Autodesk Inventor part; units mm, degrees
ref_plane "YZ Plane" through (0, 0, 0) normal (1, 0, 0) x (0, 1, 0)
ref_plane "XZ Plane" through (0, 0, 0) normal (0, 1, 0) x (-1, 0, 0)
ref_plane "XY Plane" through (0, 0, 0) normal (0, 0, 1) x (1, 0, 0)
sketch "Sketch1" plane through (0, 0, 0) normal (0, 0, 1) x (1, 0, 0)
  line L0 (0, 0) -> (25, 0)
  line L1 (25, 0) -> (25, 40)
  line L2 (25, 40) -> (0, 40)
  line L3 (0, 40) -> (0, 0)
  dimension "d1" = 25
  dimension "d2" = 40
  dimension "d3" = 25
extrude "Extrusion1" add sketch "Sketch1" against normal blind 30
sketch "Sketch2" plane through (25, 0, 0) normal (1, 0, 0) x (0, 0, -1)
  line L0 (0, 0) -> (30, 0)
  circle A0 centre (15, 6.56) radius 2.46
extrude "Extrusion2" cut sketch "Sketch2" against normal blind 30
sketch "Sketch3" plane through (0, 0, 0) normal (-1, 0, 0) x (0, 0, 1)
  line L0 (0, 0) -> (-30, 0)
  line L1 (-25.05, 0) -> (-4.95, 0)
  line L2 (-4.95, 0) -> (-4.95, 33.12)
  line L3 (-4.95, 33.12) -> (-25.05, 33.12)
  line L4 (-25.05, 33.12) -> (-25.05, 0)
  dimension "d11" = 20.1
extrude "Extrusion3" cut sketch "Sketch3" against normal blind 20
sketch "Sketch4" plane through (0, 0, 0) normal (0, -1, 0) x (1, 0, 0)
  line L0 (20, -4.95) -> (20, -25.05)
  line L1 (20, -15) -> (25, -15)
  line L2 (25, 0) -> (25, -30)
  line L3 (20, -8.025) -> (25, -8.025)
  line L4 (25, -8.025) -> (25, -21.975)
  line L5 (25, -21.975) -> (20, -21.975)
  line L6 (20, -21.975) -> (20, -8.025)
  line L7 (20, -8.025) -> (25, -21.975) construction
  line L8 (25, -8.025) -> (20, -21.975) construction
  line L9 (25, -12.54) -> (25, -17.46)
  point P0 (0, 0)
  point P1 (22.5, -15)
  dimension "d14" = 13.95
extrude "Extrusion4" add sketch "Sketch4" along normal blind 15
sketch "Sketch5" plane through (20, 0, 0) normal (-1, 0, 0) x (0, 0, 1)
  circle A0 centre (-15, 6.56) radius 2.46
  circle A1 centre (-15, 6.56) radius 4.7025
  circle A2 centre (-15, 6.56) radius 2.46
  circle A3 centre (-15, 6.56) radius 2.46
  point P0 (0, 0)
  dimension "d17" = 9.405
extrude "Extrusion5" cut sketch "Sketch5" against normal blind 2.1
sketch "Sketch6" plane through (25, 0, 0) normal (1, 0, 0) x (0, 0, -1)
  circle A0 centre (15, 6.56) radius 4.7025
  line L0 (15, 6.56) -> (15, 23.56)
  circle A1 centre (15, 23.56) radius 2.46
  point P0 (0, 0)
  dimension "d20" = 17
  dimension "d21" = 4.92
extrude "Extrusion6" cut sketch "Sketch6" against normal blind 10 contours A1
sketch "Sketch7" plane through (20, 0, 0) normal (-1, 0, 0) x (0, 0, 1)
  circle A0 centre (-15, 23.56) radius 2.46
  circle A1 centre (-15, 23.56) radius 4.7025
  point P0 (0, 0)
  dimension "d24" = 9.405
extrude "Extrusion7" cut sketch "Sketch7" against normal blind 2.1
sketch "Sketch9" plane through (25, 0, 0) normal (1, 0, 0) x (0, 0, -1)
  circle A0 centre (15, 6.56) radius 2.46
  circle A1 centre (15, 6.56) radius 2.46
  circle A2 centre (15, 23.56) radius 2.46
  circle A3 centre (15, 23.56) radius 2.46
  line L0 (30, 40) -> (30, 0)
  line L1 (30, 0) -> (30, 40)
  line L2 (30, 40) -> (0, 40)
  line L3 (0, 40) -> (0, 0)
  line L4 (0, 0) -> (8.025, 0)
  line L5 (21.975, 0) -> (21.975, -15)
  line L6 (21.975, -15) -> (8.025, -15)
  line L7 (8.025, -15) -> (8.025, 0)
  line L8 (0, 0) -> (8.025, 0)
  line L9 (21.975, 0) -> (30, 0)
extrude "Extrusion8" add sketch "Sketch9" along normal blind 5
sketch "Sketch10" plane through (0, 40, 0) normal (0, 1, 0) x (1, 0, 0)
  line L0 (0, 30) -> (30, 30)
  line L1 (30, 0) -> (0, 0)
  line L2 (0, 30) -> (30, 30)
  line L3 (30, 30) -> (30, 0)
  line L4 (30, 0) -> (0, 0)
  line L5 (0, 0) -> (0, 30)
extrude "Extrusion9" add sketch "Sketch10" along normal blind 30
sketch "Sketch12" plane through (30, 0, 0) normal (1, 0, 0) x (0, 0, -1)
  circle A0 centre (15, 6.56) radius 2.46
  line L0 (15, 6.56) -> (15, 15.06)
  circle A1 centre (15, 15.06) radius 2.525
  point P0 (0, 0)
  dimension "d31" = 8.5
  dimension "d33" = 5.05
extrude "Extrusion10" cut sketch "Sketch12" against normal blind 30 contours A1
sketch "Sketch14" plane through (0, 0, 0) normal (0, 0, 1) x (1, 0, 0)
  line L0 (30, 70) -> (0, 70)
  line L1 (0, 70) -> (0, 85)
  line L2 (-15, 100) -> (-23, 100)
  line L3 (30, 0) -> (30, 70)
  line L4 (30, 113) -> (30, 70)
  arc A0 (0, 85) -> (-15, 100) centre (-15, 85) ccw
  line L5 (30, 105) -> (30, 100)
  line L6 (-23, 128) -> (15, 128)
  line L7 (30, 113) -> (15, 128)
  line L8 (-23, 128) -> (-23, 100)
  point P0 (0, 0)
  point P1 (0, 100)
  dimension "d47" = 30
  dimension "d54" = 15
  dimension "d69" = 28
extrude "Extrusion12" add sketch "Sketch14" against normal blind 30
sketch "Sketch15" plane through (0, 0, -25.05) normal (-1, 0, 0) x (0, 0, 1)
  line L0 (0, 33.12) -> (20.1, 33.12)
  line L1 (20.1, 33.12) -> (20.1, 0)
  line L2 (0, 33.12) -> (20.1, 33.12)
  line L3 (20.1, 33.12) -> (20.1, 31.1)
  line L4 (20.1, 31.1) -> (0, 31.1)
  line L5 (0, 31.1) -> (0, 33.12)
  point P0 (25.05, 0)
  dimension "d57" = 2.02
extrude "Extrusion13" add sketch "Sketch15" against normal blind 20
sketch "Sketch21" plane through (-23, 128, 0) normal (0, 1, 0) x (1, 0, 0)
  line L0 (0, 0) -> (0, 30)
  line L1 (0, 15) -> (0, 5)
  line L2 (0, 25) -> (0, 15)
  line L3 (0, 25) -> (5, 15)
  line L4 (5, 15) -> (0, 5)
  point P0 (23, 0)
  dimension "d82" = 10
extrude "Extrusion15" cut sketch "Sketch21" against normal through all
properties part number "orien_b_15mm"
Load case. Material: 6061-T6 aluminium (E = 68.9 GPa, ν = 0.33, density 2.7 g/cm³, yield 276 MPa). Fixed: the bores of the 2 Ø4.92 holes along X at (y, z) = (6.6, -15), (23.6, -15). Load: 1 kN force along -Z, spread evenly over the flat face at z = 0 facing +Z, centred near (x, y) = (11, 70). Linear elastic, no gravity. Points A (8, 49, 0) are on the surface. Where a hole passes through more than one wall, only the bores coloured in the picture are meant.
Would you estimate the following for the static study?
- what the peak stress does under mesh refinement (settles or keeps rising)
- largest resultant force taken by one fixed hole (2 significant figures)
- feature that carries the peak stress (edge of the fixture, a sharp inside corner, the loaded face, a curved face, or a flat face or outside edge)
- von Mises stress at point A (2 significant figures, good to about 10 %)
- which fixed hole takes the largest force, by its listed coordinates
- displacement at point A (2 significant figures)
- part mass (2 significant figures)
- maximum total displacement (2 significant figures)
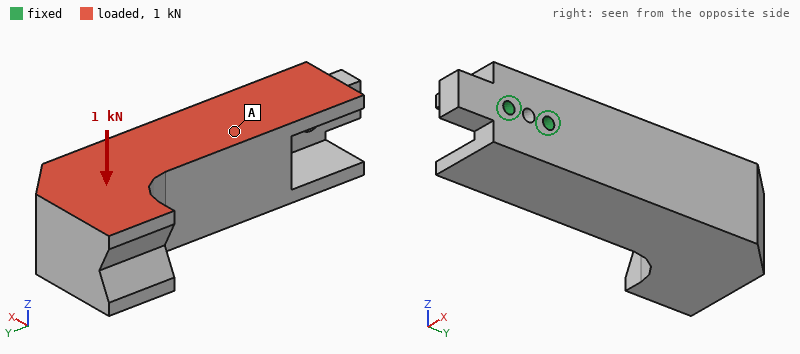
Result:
keeps rising
3.0 kN
edge of the fixture
6.7 MPa
(23.6, -15)
0.032 mm
320 g
0.12 mm
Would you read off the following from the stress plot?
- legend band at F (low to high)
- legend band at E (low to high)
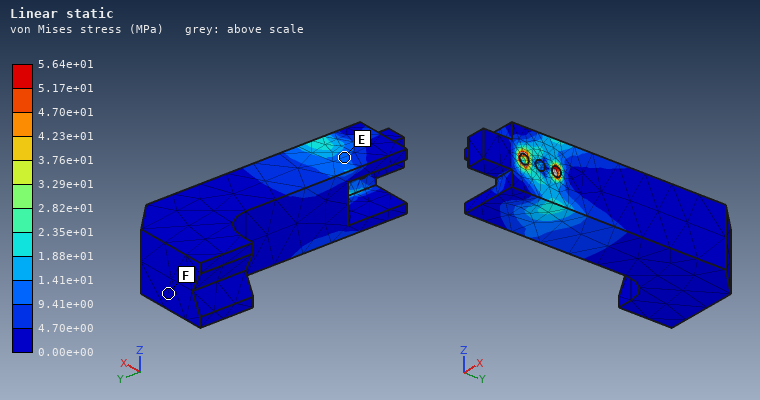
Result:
0.00e+00 to 4.70e+00 MPa
9.41e+00 to 1.41e+01 MPa
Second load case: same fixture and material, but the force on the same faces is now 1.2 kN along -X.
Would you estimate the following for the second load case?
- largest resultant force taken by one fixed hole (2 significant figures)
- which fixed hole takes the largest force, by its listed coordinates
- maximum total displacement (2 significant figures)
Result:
3.3 kN
(23.6, -15)
0.20 mm
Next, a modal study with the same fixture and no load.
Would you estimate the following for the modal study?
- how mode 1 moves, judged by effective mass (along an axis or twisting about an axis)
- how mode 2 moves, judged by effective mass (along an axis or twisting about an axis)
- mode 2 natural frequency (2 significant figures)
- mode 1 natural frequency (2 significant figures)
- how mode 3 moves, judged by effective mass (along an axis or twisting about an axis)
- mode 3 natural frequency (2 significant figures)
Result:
along X
along Z
970 Hz
830 Hz
twisting about Y
2600 Hz
